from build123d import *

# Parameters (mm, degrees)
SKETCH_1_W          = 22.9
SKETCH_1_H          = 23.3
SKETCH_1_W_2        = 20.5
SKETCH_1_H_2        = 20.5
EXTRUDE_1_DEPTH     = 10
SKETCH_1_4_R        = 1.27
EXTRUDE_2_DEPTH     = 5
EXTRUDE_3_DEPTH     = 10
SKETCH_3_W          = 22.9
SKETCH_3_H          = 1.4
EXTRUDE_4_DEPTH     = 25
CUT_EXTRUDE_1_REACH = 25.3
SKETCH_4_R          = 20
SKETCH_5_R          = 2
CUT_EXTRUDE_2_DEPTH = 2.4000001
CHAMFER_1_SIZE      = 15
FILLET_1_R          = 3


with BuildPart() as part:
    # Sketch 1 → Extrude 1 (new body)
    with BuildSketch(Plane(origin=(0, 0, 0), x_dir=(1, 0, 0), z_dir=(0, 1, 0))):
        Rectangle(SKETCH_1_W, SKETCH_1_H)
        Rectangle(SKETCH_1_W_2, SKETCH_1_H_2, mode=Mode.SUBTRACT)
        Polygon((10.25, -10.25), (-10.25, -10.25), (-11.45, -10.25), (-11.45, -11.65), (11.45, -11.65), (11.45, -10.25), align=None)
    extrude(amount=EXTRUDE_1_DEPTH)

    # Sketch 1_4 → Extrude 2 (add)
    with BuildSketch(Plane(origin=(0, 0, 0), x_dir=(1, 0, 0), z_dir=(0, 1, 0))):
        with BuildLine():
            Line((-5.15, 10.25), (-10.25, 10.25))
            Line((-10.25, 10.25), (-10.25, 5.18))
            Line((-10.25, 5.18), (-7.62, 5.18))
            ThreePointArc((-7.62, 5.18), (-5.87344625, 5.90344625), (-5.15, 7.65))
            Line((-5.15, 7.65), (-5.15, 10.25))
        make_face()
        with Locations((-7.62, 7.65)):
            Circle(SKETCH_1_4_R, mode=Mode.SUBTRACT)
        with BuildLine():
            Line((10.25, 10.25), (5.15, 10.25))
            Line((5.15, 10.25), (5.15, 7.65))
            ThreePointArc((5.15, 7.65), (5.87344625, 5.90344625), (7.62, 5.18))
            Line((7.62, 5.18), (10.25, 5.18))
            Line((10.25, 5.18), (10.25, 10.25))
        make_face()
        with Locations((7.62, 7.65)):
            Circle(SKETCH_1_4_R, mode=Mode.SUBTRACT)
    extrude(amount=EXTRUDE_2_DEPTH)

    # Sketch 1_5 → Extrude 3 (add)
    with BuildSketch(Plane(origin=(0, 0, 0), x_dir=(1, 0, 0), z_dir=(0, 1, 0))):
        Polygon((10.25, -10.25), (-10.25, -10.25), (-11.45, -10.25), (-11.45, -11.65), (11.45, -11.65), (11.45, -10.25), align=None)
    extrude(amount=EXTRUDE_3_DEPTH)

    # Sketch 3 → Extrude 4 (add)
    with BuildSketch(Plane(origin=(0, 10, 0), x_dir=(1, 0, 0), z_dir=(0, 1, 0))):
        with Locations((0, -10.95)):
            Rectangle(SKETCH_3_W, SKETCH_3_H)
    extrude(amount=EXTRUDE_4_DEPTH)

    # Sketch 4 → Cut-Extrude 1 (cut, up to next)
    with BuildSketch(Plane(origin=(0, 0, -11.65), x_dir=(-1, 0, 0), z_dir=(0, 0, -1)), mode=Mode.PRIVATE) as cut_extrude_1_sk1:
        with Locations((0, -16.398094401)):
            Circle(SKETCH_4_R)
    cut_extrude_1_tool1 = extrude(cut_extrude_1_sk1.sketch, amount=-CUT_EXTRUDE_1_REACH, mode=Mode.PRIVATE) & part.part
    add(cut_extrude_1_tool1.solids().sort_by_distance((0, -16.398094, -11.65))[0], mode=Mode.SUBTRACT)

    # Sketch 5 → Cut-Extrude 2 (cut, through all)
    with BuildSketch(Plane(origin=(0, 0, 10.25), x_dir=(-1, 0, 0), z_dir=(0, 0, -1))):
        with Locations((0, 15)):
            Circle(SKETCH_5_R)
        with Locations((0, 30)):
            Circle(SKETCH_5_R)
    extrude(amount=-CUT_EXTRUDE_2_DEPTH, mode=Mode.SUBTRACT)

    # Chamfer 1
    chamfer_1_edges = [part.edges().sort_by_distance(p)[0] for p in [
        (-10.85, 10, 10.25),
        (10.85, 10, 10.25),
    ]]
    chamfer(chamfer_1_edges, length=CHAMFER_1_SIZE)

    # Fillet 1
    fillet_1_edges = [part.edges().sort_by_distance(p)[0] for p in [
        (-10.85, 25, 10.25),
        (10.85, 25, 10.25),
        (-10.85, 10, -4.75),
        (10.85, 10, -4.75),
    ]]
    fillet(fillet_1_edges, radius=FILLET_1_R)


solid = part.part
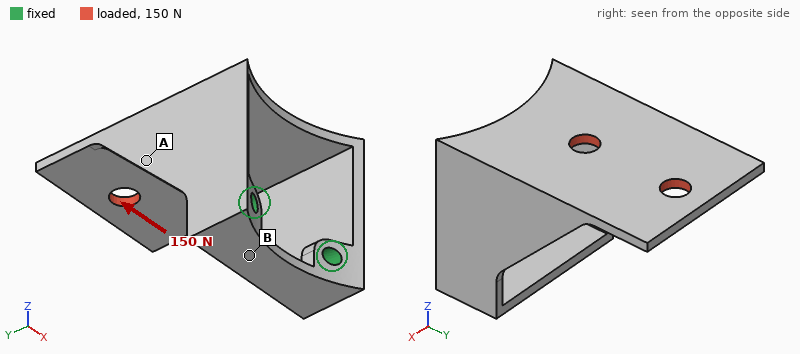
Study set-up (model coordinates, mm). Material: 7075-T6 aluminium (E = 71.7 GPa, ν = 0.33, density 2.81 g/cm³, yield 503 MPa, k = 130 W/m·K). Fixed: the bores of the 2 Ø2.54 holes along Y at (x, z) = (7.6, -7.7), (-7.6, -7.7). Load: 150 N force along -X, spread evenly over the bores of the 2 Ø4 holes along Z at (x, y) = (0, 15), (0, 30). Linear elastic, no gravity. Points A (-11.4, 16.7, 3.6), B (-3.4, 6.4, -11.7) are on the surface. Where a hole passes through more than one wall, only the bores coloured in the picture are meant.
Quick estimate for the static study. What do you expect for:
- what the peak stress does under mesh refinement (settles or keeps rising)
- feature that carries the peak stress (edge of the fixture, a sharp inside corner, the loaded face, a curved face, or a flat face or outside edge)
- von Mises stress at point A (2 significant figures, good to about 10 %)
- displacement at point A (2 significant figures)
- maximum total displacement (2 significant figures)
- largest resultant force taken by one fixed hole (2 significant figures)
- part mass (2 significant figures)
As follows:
keeps rising
edge of the fixture
88 MPa
0.30 mm
0.48 mm
140 N
5.9 g
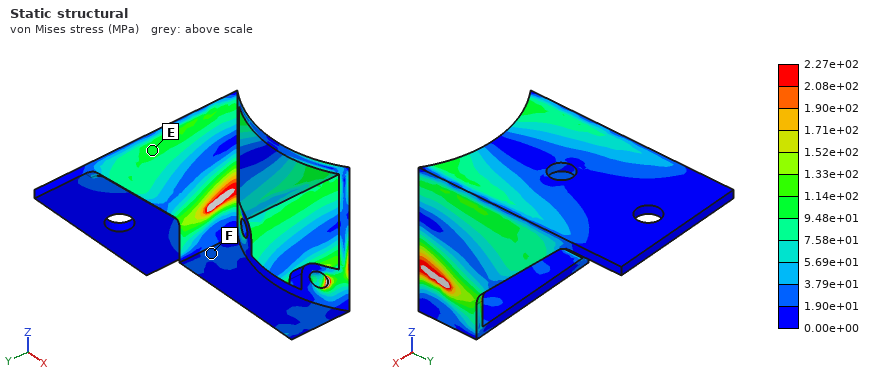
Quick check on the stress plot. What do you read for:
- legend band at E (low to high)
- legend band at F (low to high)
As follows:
9.48e+01 to 1.14e+02 MPa
1.90e+01 to 3.79e+01 MPa
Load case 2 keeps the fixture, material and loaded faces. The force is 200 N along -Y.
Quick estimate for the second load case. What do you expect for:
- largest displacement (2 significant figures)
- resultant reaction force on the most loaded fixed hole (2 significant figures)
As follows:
0.18 mm
100 N
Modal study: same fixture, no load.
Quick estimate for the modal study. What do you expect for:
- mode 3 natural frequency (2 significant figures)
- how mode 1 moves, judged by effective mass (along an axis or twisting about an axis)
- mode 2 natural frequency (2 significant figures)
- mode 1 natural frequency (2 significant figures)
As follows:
3900 Hz
along X
2700 Hz
1700 Hz
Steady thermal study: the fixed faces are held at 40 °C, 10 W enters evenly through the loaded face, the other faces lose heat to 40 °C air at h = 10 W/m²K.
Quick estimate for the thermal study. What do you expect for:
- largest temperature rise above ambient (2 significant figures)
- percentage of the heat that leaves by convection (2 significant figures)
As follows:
72 K
12 %
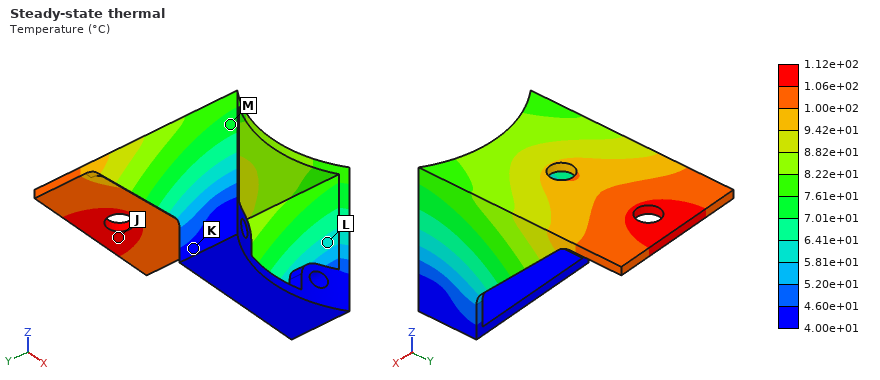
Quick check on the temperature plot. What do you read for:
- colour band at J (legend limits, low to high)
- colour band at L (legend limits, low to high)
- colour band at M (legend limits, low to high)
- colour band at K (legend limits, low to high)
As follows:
1.06e+02 to 1.12e+02 °C
5.81e+01 to 6.41e+01 °C
7.01e+01 to 7.61e+01 °C
4.00e+01 to 4.60e+01 °C
